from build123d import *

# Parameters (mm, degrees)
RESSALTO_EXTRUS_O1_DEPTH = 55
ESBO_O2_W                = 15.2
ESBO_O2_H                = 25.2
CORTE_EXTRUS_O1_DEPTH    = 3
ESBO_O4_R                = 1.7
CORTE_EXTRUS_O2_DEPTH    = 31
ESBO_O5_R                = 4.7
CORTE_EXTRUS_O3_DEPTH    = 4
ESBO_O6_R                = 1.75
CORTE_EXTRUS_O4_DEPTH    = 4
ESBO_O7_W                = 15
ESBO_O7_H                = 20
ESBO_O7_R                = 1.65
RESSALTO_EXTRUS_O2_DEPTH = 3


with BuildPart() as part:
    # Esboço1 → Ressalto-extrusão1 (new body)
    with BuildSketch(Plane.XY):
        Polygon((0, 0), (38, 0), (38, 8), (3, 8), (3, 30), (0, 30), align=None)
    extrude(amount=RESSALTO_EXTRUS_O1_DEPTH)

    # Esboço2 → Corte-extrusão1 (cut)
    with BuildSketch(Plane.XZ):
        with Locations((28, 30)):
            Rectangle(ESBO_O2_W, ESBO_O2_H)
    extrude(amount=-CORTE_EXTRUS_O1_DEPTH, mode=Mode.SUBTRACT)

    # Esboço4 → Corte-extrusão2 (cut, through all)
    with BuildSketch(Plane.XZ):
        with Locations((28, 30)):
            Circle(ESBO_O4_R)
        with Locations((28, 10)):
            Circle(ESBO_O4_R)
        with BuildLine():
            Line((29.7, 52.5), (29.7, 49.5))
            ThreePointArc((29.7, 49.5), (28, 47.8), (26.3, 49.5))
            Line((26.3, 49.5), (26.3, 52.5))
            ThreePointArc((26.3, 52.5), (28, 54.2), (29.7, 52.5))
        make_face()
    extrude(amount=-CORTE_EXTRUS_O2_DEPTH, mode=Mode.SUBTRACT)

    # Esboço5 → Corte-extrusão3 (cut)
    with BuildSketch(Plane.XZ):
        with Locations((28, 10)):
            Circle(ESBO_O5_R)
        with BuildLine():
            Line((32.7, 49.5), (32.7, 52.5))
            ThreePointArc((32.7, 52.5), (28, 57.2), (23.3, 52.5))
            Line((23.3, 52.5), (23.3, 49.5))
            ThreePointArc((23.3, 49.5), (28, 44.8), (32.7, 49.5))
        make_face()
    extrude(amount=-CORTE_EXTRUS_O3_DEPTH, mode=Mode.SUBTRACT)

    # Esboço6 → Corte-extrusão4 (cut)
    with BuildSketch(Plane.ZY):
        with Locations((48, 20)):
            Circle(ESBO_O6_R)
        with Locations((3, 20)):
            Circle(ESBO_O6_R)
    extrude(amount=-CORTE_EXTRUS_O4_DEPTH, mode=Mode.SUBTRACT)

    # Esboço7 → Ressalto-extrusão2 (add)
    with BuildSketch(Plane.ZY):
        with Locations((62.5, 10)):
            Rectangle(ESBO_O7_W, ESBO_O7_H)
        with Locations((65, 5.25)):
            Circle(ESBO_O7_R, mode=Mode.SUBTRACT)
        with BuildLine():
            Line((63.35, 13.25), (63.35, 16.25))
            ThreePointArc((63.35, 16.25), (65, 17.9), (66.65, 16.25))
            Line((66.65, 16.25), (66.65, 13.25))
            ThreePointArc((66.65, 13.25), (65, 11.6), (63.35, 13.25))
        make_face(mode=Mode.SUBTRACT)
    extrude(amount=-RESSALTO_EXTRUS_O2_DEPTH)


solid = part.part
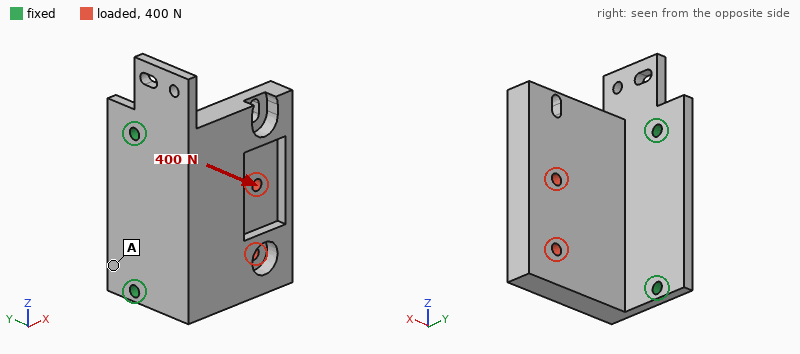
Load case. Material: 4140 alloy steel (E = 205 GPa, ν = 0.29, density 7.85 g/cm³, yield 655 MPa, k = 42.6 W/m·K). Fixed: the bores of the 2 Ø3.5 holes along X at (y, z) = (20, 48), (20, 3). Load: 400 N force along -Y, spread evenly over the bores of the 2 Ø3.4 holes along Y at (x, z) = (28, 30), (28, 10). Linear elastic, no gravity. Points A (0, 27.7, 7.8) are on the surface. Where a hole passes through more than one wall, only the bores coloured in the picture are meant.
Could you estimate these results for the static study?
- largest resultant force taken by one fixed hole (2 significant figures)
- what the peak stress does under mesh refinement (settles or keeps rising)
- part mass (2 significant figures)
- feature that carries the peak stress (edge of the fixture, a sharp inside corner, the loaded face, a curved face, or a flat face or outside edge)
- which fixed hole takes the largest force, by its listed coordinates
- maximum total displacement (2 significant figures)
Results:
250 N
keeps rising
150 g
edge of the fixture
(20, 3)
0.25 mm
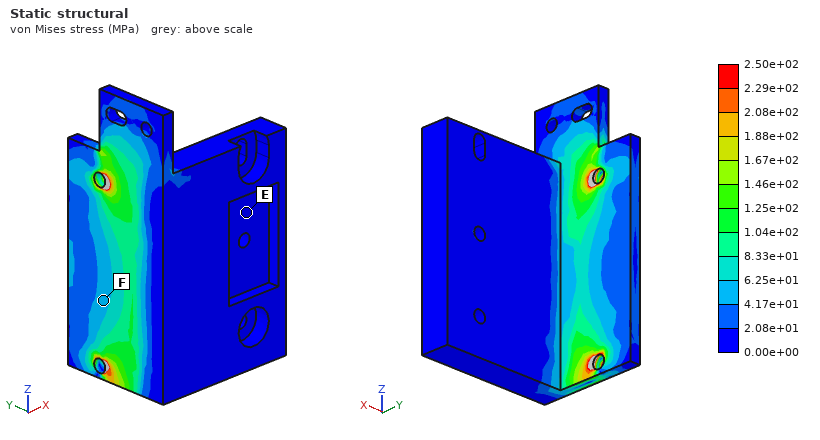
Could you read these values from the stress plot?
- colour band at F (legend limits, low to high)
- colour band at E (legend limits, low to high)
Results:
4.17e+01 to 6.25e+01 MPa
0.00e+00 to 2.08e+01 MPa
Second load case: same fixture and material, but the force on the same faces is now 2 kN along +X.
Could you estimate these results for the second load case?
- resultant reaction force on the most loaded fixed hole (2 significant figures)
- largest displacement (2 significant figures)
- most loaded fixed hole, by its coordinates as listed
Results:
1.2 kN
0.40 mm
(20, 3)
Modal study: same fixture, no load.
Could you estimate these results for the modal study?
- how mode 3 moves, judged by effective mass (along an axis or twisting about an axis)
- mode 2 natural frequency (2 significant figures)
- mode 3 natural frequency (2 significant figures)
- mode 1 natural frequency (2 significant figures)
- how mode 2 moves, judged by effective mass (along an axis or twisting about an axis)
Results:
along X
2800 Hz
4000 Hz
860 Hz
along Z
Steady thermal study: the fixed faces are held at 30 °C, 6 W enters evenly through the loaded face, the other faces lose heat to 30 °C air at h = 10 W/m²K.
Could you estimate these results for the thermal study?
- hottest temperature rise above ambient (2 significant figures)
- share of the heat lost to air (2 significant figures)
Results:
26 K
22 %
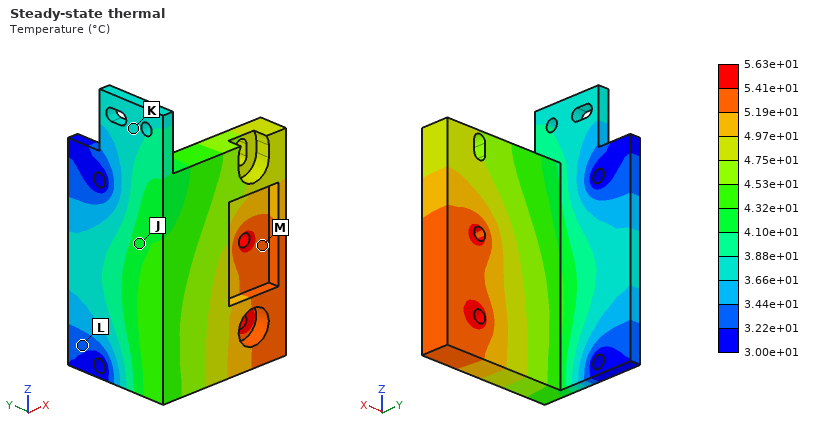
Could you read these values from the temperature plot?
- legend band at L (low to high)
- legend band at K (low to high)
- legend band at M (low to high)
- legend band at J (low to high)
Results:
3.22e+01 to 3.44e+01 °C
3.66e+01 to 3.88e+01 °C
5.19e+01 to 5.41e+01 °C
4.10e+01 to 4.32e+01 °C
